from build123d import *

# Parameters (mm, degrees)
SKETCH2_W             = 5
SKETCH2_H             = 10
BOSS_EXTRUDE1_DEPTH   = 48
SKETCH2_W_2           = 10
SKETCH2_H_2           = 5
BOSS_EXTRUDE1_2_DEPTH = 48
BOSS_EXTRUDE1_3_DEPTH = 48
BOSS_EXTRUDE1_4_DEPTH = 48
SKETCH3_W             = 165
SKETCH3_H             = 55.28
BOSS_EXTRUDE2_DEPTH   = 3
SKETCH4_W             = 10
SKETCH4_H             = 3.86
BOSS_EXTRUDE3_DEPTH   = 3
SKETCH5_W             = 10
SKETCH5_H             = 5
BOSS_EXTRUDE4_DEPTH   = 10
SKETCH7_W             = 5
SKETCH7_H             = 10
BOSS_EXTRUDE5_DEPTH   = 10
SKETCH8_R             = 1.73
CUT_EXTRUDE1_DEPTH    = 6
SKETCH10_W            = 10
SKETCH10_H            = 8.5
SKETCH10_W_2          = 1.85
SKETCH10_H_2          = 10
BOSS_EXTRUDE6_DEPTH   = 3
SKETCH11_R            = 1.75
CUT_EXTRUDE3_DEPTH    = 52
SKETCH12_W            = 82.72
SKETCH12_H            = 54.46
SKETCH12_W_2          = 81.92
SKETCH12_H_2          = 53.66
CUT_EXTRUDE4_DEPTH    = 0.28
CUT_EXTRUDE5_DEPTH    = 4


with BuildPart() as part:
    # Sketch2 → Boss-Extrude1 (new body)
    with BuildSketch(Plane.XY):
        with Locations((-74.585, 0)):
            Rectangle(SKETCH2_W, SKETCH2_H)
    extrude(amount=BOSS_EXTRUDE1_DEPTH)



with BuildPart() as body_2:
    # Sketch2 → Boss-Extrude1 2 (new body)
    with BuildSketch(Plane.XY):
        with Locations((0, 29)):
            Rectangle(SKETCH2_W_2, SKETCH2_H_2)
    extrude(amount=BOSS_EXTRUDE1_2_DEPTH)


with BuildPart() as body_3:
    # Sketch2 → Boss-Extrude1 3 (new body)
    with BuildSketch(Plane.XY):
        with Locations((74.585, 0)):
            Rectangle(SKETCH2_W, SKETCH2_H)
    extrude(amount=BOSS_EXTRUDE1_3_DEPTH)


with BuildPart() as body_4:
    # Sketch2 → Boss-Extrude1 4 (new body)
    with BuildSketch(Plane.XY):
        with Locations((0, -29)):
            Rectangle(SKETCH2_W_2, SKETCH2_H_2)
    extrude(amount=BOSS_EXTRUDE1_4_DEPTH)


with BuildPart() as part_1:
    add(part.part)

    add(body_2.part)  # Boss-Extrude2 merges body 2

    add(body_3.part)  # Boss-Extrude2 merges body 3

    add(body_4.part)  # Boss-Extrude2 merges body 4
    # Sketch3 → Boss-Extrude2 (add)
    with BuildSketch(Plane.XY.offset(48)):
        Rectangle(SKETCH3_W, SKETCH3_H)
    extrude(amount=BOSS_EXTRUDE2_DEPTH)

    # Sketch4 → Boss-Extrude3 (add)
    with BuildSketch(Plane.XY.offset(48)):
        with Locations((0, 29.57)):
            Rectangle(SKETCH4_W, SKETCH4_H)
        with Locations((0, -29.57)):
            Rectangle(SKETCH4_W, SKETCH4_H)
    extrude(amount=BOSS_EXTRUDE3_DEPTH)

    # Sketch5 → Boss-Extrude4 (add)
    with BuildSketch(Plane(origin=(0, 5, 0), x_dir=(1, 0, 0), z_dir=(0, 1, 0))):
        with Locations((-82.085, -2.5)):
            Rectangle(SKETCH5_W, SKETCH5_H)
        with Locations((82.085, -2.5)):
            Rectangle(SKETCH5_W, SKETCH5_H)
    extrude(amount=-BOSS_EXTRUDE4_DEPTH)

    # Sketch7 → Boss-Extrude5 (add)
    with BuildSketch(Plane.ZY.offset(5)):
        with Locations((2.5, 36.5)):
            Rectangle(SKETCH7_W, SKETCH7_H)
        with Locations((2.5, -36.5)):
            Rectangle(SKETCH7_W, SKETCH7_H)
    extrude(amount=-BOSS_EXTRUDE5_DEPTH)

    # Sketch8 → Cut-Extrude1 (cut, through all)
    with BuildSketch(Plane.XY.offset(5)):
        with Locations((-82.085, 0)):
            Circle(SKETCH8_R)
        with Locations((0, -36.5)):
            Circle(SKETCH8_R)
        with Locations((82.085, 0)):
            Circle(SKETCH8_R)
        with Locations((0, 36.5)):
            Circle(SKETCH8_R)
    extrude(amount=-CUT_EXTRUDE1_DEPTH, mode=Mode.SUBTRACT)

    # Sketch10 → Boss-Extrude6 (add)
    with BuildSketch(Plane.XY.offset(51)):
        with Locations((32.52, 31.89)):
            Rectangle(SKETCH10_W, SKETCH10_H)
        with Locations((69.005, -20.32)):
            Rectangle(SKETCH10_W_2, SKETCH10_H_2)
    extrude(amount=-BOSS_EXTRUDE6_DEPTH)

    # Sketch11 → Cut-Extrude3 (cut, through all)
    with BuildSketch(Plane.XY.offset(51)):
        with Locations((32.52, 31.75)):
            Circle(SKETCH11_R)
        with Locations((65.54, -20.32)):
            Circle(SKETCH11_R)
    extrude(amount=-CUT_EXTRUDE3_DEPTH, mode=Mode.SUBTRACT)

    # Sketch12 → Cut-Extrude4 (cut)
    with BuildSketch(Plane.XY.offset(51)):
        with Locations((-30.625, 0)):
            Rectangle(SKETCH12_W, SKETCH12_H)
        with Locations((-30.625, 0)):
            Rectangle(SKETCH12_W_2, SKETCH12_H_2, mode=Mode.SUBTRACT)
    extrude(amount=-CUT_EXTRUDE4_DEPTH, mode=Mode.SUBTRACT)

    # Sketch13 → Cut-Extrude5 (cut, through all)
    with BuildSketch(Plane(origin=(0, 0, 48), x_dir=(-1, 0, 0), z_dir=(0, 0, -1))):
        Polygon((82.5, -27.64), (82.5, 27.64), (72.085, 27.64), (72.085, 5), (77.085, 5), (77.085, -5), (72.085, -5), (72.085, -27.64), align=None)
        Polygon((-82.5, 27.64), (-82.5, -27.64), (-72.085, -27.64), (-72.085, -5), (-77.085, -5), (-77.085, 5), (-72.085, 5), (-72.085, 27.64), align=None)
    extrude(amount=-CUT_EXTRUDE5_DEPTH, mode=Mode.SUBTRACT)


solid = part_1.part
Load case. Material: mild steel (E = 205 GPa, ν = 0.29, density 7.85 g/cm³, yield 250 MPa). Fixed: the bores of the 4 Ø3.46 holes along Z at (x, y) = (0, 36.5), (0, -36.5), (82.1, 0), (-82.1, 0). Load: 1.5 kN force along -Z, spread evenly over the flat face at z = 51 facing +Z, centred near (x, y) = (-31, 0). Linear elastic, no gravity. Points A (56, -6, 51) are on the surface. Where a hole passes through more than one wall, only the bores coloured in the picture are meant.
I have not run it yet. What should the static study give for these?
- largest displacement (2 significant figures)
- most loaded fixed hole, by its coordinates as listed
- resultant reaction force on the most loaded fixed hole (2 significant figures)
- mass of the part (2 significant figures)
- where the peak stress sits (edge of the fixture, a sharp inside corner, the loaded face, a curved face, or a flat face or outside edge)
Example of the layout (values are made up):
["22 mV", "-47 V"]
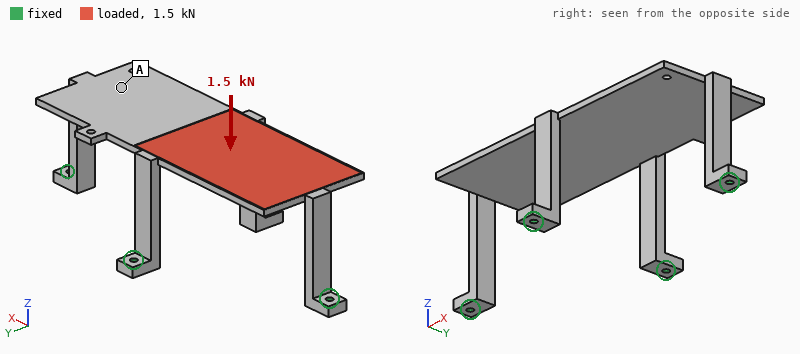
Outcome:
["0.14 mm", "(-82.1, 0)", "600 N", "280 g", "a flat face or outside edge"]
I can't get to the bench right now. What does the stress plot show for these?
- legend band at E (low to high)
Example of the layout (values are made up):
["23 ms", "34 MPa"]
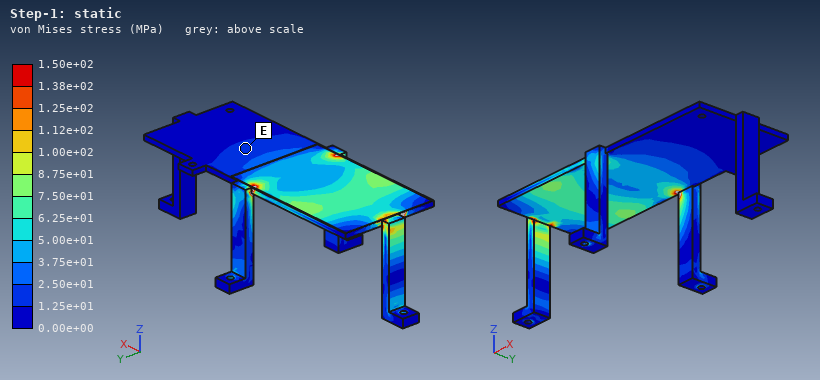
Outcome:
["1.25e+01 to 2.50e+01 MPa"]
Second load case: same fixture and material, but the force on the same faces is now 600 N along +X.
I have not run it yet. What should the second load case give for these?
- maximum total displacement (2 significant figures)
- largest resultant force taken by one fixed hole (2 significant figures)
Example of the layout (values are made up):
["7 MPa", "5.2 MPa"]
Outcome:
["0.11 mm", "190 N"]
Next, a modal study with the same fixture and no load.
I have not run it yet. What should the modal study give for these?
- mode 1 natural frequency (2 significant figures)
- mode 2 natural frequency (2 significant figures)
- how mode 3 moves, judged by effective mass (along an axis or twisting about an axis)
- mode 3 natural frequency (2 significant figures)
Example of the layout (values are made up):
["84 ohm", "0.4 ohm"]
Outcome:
["780 Hz", "810 Hz", "twisting about Z", "1100 Hz"]
